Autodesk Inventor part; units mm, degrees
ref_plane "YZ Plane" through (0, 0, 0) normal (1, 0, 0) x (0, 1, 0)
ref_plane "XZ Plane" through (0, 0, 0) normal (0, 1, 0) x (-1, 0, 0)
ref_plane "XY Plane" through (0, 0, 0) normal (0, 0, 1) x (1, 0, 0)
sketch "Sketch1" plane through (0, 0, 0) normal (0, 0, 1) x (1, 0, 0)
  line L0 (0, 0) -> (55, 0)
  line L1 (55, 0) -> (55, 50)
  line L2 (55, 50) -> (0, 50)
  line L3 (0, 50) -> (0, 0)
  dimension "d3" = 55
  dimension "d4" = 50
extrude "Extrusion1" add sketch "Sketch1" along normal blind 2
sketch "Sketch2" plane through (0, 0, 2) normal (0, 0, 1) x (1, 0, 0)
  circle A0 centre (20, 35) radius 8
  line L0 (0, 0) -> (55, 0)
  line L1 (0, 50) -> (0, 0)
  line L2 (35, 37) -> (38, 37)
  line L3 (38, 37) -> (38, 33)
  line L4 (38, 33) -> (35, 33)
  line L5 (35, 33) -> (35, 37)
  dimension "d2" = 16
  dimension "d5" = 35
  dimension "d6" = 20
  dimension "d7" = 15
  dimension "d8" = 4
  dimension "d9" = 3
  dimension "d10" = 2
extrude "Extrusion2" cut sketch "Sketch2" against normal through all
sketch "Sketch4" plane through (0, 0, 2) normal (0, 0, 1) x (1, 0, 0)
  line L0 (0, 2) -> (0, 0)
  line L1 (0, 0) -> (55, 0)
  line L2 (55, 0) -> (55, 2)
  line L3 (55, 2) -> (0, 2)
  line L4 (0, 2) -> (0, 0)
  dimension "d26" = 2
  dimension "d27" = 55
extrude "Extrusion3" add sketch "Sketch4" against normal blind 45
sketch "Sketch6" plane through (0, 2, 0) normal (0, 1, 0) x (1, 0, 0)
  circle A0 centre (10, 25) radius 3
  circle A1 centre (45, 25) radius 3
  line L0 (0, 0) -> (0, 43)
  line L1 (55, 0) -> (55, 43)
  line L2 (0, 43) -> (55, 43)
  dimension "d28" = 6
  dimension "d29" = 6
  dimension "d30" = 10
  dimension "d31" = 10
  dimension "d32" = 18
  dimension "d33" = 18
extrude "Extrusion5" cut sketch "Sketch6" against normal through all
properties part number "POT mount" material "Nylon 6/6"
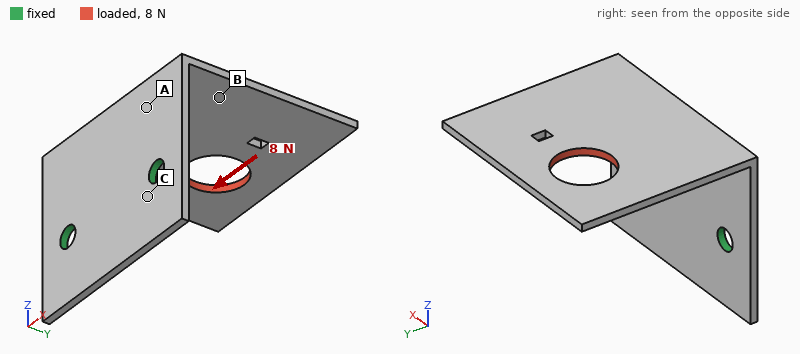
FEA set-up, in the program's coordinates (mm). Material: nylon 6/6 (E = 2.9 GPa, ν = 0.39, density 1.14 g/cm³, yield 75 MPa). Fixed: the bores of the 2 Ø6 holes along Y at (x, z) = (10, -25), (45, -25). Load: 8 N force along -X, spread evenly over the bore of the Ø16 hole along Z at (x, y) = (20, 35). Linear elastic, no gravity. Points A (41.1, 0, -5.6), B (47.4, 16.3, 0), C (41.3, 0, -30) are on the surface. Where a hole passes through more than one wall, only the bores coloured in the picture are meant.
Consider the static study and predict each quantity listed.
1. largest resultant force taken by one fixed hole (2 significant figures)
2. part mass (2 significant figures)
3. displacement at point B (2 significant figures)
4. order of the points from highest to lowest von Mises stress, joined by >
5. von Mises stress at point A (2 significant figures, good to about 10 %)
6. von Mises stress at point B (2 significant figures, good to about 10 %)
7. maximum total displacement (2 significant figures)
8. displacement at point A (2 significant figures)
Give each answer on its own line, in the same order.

9.7 N
11 g
0.39 mm
A > B > C
2.7 MPa
1.3 MPa
0.88 mm
0.14 mm
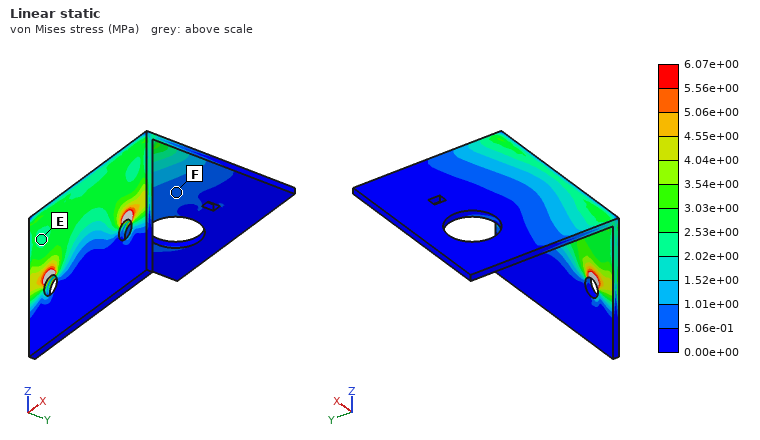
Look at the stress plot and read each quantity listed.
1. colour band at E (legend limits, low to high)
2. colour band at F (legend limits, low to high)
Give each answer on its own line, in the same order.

2.02e+00 to 2.53e+00 MPa
5.06e-01 to 1.01e+00 MPa
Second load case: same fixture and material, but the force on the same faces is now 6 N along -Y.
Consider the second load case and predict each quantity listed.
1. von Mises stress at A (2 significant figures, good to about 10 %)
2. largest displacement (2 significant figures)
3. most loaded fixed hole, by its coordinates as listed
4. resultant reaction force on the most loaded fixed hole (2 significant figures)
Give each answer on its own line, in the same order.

1.00 MPa
0.90 mm
(10, -25)
4.2 N
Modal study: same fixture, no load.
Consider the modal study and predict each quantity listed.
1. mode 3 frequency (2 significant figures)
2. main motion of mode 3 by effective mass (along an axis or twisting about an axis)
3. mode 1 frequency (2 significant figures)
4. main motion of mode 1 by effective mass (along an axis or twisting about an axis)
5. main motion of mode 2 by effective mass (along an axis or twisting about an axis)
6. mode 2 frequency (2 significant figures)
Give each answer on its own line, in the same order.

430 Hz
along Y
130 Hz
along Z
along X
260 Hz
